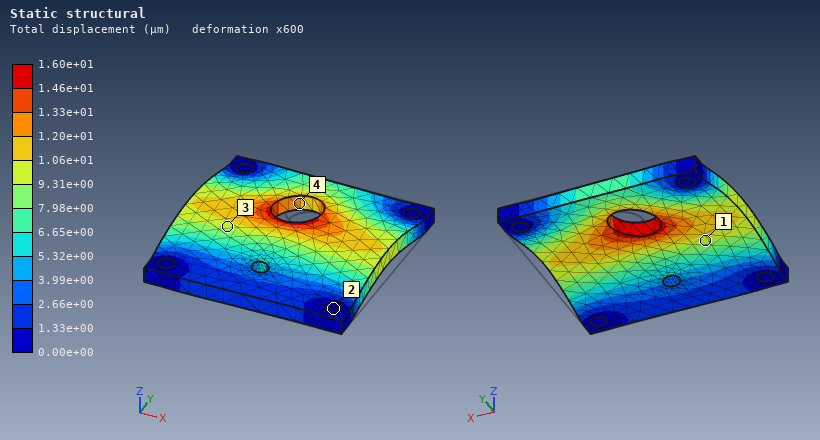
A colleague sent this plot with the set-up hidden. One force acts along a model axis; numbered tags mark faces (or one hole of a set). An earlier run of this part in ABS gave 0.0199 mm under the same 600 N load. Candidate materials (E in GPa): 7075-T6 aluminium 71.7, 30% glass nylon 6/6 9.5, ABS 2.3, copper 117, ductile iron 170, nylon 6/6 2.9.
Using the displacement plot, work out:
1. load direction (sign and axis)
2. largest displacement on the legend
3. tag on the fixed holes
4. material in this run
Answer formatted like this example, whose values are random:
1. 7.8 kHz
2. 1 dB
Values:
1. -X
2. 1.60e+01 µm
3. 2
4. nylon 6/6
